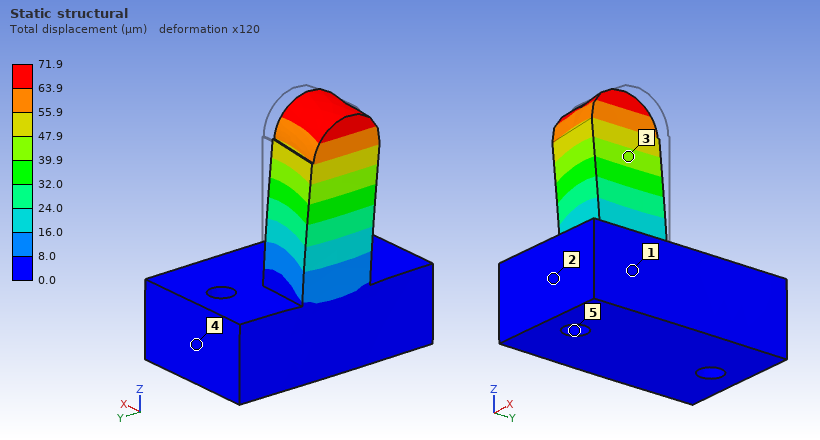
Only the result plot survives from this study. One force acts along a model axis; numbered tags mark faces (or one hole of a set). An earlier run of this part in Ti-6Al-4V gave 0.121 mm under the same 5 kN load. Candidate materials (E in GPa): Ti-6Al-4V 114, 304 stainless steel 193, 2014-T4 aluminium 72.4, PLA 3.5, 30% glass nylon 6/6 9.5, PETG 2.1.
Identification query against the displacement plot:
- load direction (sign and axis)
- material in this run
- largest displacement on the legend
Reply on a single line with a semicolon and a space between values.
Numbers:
-X; 304 stainless steel; 71.9 µm
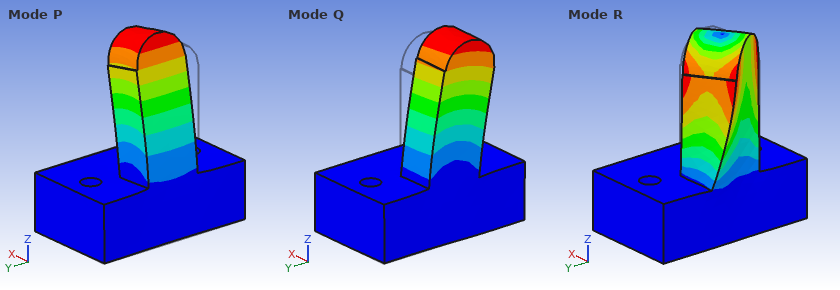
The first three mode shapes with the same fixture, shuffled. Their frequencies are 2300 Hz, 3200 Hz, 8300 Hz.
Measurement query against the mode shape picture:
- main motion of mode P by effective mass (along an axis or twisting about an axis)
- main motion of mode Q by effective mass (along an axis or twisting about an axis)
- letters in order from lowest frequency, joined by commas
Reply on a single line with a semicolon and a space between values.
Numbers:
along X; along Y; P, Q, R
